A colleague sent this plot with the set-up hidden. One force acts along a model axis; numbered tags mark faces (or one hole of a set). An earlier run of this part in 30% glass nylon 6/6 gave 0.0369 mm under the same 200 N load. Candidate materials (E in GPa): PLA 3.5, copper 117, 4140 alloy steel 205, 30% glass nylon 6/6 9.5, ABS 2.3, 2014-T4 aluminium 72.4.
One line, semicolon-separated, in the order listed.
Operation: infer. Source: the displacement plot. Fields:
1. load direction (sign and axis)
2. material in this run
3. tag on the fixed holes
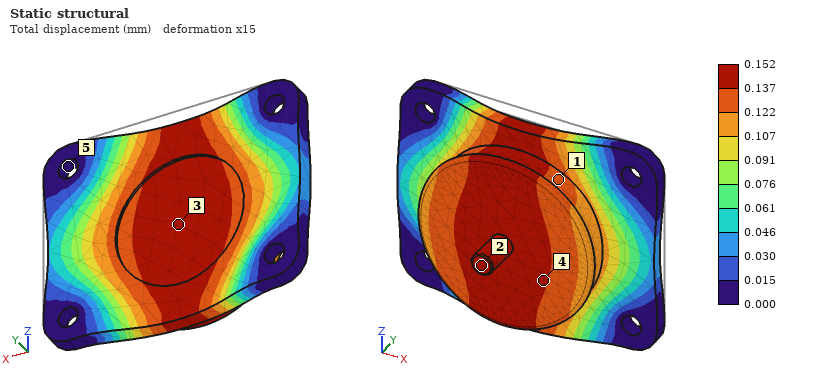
-Y; ABS; 5
